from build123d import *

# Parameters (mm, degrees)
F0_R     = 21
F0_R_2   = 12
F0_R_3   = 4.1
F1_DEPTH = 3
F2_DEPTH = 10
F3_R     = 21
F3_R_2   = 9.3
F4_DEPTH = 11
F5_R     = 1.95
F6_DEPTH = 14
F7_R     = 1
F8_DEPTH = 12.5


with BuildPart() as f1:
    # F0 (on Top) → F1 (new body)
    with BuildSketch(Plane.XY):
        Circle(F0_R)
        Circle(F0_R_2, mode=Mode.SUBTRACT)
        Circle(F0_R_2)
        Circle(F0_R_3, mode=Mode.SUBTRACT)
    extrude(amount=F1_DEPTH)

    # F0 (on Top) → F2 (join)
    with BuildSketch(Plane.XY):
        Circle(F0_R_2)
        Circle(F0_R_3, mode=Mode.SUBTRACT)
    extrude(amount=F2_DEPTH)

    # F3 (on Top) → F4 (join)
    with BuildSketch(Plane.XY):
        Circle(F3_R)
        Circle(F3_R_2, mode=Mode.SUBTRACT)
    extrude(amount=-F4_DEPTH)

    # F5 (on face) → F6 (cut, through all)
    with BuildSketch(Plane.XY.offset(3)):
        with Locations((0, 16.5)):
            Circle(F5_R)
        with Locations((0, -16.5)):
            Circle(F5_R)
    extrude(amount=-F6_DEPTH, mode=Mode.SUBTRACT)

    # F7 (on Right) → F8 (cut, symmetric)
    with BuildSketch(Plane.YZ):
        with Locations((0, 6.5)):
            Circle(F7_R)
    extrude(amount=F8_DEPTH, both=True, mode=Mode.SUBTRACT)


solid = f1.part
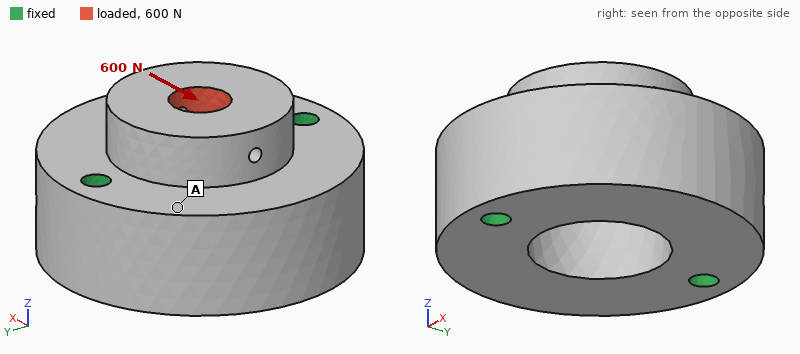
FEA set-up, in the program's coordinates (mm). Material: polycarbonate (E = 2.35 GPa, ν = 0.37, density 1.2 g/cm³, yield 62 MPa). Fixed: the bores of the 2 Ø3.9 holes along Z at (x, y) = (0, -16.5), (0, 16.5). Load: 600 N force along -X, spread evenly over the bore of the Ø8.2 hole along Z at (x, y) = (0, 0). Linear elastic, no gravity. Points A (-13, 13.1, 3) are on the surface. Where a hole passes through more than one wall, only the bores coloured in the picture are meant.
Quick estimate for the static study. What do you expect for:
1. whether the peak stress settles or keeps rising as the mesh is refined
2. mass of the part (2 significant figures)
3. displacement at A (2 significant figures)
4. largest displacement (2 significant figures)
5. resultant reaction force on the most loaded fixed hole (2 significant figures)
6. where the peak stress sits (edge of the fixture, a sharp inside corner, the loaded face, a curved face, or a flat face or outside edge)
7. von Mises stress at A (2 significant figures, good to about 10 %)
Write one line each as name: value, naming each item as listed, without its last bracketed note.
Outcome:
whether the peak stress settles or keeps rising as the mesh is refined: keeps rising
mass of the part: 22 g
displacement at A: 33 µm
largest displacement: 63 µm
resultant reaction force on the most loaded fixed hole: 300 N
where the peak stress sits: edge of the fixture
von Mises stress at A: 1.7 MPa
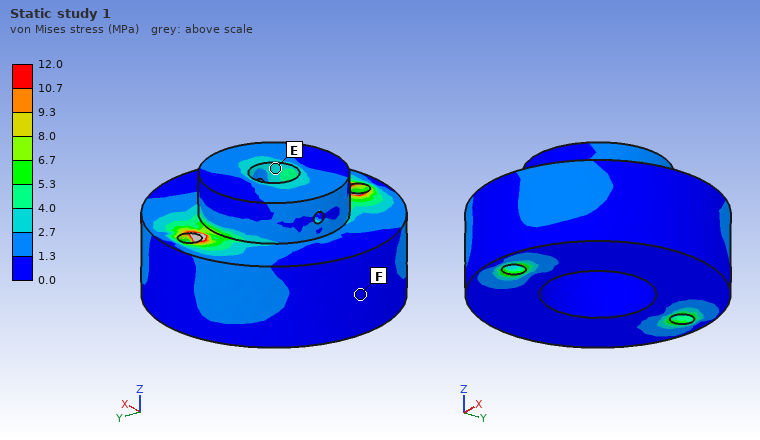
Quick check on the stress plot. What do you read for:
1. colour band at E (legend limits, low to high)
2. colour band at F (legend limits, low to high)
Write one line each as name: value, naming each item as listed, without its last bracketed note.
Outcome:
colour band at E: 2.7 to 4.0 MPa
colour band at F: 0.0 to 1.3 MPa
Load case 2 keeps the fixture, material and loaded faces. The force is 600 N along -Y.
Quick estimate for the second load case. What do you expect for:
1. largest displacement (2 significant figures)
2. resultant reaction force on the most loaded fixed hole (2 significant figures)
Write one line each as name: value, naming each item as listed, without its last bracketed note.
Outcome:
largest displacement: 31 µm
resultant reaction force on the most loaded fixed hole: 330 N
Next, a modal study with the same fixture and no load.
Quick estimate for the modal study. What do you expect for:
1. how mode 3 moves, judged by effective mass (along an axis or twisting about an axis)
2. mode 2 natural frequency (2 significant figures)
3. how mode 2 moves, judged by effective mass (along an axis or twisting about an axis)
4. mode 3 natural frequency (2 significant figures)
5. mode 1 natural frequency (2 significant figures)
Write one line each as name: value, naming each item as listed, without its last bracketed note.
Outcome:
how mode 3 moves, judged by effective mass: twisting about Z
mode 2 natural frequency: 5700 Hz
how mode 2 moves, judged by effective mass: along Z
mode 3 natural frequency: 8200 Hz
mode 1 natural frequency: 4300 Hz
